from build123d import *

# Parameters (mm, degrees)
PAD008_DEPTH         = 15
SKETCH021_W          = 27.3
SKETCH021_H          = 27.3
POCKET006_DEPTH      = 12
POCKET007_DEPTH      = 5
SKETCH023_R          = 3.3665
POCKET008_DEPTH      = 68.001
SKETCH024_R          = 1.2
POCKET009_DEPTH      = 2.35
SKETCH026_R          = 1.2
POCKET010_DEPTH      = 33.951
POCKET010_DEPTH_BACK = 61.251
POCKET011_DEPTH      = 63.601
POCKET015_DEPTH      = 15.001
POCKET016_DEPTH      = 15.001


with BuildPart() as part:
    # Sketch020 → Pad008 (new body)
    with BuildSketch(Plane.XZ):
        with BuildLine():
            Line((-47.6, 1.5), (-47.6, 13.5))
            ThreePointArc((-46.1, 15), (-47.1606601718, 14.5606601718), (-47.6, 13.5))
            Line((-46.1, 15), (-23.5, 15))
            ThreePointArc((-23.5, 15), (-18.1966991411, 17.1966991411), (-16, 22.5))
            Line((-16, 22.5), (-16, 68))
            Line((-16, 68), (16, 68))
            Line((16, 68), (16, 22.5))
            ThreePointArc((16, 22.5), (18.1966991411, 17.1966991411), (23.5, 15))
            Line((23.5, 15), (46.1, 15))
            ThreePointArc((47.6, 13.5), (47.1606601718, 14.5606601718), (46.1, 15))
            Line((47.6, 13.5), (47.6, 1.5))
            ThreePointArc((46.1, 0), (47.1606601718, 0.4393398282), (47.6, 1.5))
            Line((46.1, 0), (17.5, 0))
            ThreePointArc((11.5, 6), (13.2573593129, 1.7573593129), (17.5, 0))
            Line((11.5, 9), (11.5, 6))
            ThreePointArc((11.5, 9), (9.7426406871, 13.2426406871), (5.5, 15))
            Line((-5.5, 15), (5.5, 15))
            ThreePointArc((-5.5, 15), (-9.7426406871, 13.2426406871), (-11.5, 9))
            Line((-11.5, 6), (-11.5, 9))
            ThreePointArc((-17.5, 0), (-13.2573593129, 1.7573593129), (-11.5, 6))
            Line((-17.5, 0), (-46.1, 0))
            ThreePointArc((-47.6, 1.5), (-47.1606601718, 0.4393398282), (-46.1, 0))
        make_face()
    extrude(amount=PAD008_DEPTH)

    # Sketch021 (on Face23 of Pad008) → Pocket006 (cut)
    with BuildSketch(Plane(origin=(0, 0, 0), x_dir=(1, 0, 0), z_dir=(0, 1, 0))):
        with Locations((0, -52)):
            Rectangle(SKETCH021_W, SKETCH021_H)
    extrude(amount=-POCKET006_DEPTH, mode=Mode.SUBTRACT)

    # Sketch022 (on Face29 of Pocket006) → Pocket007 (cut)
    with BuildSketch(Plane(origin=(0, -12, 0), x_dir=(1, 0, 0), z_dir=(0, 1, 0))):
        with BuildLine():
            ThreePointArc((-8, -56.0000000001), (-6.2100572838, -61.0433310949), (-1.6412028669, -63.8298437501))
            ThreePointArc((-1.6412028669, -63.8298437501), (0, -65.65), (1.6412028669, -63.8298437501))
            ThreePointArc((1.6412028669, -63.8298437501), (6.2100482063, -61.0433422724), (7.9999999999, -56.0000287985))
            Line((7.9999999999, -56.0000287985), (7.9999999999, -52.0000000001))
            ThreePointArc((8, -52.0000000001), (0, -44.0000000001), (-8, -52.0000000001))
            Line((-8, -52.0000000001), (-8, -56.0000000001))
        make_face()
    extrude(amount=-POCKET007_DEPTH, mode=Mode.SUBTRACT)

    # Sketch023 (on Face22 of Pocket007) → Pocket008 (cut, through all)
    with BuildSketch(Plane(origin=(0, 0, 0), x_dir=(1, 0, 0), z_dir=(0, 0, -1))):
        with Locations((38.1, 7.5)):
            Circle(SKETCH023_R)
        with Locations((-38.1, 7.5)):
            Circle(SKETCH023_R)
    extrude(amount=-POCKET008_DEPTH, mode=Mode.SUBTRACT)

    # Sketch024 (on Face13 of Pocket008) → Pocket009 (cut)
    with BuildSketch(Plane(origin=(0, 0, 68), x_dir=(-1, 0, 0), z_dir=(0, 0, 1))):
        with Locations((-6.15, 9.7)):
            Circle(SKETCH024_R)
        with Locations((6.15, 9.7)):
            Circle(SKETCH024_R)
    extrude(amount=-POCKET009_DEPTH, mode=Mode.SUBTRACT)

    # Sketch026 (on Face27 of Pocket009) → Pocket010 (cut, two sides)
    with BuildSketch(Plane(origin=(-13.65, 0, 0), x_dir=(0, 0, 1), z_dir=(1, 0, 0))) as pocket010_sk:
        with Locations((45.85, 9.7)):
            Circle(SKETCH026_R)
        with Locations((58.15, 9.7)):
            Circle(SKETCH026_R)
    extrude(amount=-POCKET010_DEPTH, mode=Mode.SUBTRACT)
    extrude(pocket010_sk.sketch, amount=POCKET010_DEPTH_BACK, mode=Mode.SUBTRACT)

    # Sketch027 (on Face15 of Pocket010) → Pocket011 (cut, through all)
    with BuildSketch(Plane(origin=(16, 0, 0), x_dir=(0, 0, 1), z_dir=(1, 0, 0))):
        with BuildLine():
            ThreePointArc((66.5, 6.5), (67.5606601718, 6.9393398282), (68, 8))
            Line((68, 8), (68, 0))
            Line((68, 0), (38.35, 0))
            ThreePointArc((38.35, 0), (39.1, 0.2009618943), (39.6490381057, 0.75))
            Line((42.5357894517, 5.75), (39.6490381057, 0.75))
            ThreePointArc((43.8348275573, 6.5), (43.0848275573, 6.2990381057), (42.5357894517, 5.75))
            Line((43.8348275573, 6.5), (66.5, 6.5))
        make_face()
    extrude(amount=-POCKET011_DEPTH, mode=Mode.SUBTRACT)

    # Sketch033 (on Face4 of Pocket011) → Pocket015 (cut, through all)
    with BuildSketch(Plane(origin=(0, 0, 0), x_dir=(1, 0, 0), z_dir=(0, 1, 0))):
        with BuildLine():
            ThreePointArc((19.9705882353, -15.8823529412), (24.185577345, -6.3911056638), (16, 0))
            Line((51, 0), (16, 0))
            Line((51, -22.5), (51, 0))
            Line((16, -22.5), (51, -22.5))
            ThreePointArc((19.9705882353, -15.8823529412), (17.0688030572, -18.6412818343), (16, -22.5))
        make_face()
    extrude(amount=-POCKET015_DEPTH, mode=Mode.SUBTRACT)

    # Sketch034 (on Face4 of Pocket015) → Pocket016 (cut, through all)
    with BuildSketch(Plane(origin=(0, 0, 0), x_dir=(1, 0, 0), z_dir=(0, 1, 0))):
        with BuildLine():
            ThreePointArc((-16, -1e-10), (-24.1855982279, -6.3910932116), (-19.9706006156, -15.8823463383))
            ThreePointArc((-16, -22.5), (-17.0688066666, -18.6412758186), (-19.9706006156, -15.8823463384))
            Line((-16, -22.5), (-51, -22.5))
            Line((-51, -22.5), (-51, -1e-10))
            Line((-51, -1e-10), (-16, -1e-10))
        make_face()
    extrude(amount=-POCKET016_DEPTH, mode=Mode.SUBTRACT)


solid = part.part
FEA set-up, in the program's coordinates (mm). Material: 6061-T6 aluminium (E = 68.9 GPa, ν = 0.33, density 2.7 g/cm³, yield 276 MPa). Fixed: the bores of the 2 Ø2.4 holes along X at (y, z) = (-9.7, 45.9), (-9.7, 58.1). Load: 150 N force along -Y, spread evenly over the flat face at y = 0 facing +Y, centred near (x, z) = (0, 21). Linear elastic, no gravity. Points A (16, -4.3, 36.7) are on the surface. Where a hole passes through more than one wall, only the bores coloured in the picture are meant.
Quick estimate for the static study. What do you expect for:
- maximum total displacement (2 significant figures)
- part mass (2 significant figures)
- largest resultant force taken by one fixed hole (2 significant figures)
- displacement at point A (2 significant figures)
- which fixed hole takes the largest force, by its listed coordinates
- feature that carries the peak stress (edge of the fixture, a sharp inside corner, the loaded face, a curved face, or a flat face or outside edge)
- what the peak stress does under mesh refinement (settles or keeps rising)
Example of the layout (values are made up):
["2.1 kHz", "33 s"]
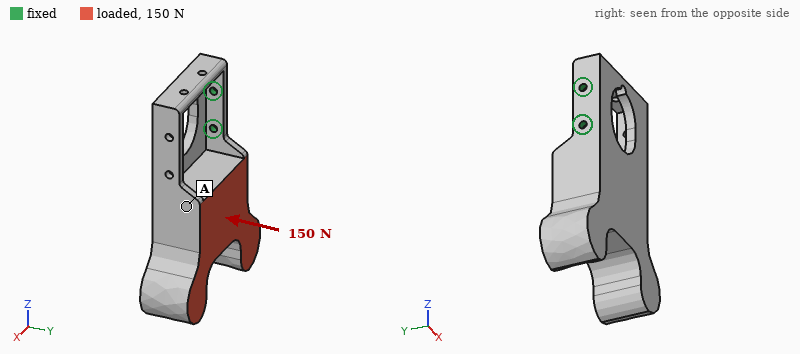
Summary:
["0.32 mm", "54 g", "420 N", "0.19 mm", "(-9.7, 45.9)", "edge of the fixture", "keeps rising"]
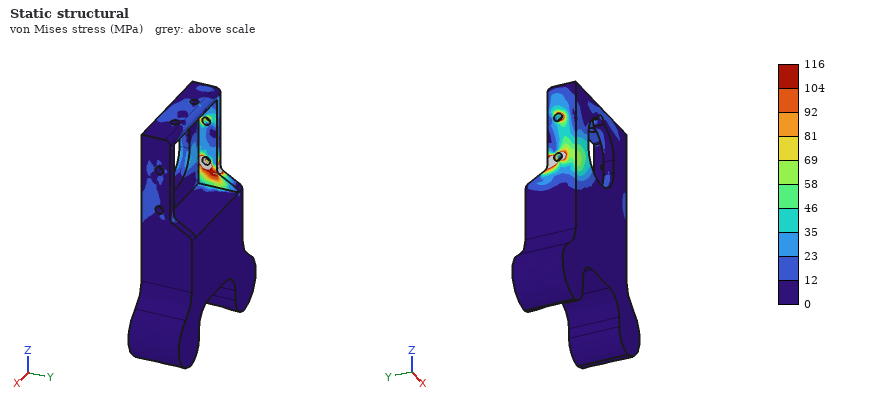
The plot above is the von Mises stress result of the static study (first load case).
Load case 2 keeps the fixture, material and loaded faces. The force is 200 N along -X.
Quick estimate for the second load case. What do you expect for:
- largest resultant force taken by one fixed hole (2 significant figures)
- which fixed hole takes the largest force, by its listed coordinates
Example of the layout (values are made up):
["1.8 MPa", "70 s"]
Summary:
["500 N", "(-9.7, 45.9)"]
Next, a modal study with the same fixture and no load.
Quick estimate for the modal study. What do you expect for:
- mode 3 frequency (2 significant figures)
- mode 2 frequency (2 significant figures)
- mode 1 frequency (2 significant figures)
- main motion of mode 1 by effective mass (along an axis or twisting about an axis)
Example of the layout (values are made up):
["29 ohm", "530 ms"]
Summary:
["1700 Hz", "1100 Hz", "640 Hz", "along Y"]
